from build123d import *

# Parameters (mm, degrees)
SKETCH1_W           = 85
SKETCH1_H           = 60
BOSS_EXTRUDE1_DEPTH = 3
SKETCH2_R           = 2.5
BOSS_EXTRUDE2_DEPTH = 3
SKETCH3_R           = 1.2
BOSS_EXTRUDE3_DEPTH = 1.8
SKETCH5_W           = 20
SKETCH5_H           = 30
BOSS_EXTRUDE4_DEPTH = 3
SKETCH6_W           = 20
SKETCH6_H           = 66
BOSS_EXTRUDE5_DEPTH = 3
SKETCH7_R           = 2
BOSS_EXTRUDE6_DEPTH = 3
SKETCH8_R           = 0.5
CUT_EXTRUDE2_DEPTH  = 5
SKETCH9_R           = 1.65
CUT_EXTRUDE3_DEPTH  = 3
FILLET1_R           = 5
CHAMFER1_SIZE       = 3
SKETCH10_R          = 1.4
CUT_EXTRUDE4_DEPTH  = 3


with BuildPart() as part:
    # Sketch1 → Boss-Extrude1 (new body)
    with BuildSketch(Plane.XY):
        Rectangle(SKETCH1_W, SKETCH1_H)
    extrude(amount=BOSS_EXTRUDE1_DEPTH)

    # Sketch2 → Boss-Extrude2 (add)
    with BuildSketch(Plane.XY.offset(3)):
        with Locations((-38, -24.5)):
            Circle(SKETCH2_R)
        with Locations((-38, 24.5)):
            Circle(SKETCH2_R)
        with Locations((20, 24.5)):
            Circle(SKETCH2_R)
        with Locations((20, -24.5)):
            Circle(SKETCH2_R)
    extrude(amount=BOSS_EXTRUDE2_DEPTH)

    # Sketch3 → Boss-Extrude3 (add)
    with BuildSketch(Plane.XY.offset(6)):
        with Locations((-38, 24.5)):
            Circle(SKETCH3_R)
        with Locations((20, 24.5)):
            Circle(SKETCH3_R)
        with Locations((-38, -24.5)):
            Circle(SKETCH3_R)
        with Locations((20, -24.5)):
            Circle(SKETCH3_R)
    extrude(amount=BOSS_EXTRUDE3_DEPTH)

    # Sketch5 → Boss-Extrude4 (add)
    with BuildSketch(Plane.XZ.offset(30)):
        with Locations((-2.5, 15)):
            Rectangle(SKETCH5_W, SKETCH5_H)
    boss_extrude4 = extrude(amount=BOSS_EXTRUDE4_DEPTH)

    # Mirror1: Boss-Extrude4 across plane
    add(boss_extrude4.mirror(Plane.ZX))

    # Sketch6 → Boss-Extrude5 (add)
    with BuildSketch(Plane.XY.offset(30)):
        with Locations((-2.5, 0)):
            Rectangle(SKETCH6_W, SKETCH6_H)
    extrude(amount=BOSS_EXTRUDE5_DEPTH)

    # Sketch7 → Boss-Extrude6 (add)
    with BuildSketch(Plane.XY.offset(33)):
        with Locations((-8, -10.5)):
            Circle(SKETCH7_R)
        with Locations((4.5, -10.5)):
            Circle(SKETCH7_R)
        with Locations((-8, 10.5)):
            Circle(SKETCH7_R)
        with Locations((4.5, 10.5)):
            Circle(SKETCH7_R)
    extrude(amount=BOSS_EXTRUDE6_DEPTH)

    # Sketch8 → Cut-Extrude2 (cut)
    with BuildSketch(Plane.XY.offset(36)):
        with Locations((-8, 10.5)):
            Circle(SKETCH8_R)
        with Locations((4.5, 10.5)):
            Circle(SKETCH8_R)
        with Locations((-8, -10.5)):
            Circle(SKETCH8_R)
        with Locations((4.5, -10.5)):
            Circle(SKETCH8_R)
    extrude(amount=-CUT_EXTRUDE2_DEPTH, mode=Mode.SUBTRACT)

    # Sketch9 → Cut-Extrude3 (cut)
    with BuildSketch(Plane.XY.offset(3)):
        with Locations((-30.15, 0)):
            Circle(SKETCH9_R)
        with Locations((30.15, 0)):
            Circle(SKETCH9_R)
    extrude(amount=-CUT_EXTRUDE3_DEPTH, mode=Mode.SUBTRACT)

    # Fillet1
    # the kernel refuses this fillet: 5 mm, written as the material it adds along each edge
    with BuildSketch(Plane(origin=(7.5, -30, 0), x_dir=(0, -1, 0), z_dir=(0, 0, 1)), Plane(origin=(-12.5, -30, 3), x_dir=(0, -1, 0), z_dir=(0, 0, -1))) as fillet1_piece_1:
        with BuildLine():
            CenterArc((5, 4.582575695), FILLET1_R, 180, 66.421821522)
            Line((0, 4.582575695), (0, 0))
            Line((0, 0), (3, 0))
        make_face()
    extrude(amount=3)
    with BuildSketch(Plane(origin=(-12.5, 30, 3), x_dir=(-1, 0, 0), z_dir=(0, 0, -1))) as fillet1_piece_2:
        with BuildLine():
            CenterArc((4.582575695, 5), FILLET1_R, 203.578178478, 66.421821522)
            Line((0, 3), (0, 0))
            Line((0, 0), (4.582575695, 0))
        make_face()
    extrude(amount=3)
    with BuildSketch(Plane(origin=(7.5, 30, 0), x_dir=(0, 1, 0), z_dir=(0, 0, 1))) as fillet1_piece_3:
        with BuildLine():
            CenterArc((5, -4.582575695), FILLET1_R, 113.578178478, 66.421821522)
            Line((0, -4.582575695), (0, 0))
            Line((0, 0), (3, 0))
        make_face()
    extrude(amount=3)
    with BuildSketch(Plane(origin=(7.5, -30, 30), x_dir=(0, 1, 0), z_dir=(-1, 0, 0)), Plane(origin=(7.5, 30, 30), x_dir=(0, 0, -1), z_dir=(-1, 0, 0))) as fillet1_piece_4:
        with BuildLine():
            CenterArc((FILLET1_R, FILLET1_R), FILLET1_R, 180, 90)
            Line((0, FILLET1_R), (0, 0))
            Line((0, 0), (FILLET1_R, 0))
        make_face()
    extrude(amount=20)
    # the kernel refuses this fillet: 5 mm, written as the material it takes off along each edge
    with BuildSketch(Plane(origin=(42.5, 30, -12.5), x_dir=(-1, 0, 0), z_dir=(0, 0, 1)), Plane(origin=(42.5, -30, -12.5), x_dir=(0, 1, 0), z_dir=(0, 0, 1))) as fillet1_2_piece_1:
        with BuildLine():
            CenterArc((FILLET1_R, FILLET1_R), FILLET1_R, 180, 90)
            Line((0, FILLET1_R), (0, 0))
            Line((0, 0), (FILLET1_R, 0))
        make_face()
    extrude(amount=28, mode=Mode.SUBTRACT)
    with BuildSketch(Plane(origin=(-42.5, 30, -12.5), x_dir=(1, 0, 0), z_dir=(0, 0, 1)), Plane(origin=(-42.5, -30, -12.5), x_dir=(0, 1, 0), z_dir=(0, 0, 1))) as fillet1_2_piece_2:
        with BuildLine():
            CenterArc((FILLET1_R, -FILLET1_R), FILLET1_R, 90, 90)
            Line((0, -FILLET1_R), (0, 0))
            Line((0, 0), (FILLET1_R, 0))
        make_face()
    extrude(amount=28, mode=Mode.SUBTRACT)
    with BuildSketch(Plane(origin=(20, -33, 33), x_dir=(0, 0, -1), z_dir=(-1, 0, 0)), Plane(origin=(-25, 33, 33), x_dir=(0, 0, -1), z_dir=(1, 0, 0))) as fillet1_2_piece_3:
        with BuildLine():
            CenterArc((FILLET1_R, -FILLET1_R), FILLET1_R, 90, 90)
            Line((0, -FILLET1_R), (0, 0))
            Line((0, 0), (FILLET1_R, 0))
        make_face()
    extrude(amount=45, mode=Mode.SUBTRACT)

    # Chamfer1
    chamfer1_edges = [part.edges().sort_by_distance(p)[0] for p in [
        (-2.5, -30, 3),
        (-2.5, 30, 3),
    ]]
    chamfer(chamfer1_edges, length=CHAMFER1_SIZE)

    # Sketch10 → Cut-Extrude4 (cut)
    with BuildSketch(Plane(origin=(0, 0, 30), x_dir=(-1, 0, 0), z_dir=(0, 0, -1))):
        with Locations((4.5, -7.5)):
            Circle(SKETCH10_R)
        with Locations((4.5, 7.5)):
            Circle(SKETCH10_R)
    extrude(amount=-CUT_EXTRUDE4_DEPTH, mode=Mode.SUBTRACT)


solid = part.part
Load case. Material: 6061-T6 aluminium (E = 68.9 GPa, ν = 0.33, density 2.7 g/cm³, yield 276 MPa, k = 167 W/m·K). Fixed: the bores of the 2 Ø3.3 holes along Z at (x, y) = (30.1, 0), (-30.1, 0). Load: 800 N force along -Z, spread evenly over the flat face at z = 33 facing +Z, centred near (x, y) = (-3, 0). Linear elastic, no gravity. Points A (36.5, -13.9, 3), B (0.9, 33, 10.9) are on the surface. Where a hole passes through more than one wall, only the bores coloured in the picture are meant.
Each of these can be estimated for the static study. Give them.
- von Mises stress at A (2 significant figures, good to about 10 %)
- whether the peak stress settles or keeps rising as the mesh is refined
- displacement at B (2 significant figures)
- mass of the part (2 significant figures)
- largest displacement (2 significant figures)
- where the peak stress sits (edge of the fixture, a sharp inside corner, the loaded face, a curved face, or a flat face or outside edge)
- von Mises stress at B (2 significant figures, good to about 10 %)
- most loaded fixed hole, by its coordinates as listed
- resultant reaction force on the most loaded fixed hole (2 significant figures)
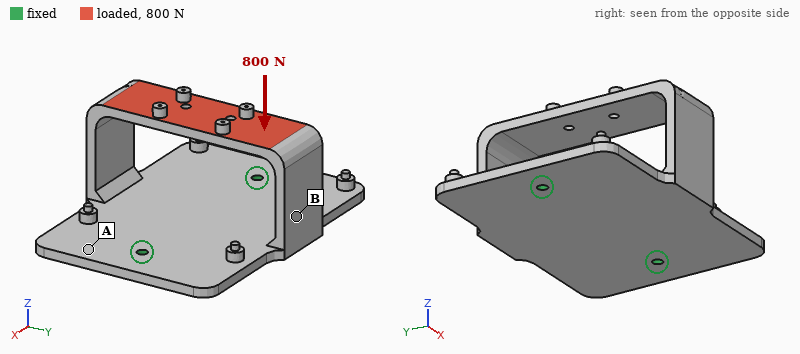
39 MPa
keeps rising
0.37 mm
63 g
0.69 mm
edge of the fixture
80 MPa
(-30.1, 0)
440 N
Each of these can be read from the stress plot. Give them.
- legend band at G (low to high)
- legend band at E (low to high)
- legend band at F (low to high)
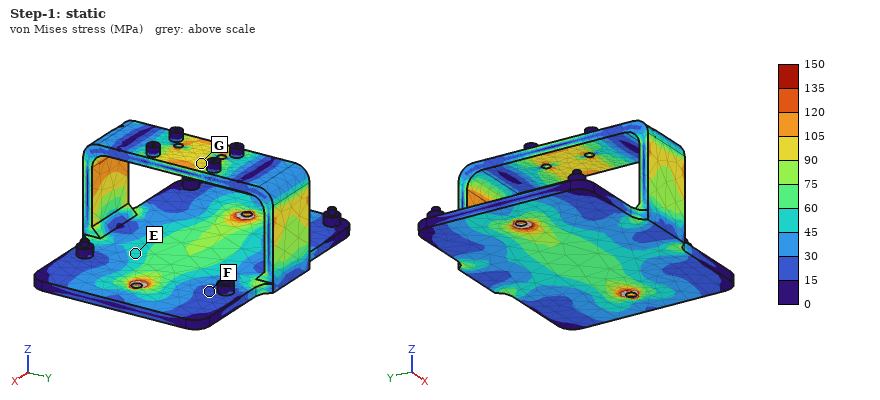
90 to 105 MPa
45 to 60 MPa
15 to 30 MPa
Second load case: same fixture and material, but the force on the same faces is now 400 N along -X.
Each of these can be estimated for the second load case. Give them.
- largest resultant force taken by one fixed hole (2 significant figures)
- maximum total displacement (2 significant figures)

320 N
0.37 mm
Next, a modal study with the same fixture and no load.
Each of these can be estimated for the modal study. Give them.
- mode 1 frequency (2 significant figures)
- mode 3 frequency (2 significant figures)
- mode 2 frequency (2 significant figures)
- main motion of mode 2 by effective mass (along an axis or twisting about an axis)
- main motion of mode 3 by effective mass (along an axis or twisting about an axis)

800 Hz
1500 Hz
1400 Hz
along Z
along X
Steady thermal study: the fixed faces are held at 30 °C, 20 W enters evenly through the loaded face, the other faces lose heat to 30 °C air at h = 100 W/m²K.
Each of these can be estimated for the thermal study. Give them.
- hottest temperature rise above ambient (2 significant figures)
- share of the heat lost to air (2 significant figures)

34 K
68 %
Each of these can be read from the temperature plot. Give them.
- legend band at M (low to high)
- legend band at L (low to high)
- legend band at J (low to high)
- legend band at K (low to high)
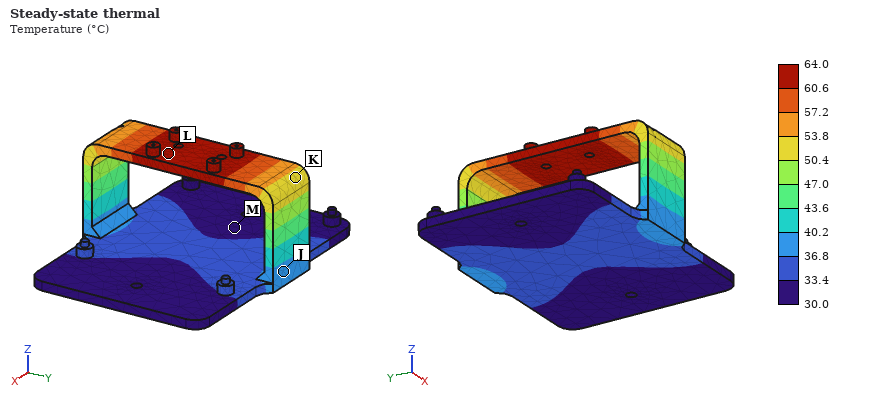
30.0 to 33.4 °C
60.6 to 64.0 °C
36.8 to 40.2 °C
50.4 to 53.8 °C
